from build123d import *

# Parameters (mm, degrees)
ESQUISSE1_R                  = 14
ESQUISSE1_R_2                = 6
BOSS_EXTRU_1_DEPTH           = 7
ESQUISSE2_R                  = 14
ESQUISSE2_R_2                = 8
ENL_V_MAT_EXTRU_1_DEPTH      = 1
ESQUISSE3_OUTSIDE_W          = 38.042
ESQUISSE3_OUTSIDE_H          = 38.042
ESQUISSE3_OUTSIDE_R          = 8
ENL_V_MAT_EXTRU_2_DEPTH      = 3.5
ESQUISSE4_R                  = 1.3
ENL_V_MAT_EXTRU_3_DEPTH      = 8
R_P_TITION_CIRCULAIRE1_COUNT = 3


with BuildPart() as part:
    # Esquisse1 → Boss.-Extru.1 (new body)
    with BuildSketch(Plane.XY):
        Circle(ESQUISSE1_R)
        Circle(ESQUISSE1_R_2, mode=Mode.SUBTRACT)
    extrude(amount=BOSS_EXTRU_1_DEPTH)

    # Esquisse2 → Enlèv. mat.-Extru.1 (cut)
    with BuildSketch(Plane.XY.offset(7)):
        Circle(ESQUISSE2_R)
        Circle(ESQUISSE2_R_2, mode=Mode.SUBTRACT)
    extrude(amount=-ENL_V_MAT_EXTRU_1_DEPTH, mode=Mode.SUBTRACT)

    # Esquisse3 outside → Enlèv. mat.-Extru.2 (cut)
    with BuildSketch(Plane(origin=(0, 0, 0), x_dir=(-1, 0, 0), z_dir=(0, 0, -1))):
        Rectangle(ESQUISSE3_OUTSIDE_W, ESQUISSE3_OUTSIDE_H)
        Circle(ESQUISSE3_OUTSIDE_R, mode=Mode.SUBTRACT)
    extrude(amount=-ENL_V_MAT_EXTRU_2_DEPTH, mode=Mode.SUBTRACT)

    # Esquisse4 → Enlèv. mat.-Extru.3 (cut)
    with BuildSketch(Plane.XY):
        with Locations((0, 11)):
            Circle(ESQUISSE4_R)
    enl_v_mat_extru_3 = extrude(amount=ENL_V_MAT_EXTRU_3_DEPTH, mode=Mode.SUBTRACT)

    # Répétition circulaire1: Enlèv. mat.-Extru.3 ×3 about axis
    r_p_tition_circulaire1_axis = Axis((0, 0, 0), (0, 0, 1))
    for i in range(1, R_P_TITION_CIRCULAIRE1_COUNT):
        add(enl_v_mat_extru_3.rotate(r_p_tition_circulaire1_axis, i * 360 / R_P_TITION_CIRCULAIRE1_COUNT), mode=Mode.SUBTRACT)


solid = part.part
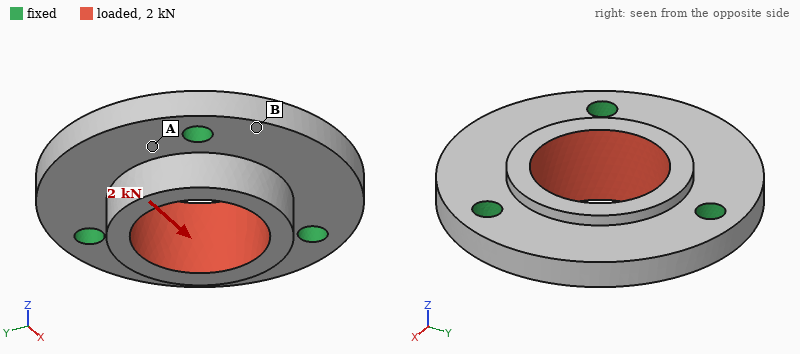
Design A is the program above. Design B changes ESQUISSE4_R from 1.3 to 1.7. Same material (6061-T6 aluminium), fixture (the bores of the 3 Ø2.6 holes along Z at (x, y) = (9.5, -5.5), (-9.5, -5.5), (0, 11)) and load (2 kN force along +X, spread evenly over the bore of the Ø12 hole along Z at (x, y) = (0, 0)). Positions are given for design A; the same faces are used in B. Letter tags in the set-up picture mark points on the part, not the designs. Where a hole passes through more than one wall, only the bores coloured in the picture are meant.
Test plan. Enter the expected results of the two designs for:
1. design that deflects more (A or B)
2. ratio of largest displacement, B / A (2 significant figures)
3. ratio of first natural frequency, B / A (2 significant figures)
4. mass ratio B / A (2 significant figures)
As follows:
A
0.89
1.1
0.98
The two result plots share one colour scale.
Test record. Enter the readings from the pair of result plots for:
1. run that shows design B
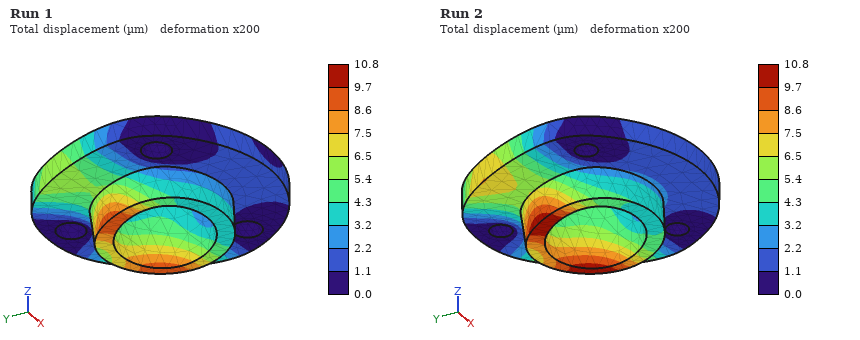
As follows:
Run 1
